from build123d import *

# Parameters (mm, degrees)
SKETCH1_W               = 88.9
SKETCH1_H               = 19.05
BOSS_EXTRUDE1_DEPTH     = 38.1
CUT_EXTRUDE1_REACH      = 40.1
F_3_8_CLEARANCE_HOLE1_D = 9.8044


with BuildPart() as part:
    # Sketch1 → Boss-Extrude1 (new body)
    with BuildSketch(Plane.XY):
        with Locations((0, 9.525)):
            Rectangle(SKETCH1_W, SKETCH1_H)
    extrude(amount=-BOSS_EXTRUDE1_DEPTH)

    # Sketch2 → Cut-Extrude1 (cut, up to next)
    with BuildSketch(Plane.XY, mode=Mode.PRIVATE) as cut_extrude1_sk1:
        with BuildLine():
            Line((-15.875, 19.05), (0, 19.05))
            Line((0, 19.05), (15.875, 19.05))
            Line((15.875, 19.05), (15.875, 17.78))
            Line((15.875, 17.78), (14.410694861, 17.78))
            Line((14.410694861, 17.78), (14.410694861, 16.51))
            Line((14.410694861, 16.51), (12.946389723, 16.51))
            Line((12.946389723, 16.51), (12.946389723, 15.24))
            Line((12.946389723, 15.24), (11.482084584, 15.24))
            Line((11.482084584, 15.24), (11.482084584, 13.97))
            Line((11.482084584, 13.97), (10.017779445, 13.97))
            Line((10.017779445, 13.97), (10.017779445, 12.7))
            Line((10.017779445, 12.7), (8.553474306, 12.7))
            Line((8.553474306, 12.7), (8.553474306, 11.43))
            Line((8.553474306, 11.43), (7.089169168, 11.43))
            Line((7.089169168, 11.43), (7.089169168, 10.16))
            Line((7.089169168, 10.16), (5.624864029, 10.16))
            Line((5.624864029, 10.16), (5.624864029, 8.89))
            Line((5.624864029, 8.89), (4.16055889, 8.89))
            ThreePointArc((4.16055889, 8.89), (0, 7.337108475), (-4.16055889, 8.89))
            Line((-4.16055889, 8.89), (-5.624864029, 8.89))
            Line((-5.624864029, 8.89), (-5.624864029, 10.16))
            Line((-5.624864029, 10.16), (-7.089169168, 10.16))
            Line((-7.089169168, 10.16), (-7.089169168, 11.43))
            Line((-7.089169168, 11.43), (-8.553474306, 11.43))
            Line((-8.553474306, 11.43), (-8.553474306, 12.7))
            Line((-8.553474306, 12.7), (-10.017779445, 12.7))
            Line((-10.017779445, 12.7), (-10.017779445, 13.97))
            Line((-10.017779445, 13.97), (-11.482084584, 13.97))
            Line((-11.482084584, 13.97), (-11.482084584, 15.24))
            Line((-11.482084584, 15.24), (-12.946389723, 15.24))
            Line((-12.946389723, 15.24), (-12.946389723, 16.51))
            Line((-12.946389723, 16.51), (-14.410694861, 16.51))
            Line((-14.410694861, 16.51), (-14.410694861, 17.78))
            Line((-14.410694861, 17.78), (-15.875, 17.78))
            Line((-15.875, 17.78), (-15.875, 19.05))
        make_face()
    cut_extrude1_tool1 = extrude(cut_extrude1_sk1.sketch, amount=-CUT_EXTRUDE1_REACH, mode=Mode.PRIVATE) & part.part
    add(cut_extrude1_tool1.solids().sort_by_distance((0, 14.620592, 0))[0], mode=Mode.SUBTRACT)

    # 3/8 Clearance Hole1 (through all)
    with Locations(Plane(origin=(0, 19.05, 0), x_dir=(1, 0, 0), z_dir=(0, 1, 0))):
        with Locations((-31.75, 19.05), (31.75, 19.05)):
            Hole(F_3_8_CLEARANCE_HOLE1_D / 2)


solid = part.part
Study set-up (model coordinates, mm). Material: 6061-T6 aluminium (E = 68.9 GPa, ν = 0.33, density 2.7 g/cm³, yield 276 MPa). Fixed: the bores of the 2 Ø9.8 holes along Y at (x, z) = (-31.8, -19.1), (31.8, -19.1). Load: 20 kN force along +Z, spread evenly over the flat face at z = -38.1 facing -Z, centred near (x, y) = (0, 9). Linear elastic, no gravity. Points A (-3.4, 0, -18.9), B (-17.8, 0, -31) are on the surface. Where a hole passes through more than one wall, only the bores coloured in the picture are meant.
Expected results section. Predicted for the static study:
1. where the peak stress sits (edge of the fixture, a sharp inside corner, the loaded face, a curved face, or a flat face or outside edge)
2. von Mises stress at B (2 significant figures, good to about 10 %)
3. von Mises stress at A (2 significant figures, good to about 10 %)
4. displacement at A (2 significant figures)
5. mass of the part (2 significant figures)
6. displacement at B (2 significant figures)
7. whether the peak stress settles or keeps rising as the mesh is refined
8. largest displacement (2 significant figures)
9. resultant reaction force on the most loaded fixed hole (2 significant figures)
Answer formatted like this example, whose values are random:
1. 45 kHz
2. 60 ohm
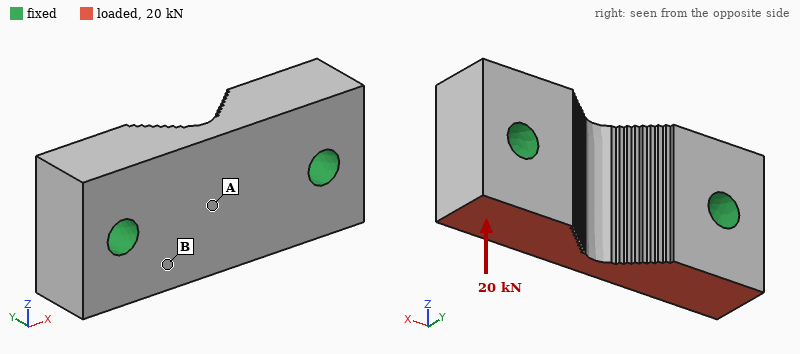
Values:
1. edge of the fixture
2. 18 MPa
3. 8.0 MPa
4. 12 µm
5. 140 g
6. 8.4 µm
7. keeps rising
8. 15 µm
9. 10 kN
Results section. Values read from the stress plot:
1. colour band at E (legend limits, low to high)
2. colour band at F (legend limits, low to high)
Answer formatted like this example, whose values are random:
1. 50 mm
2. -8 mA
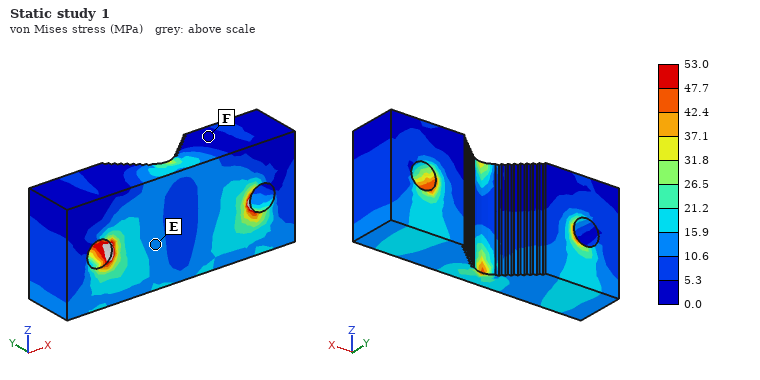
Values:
1. 10.6 to 15.9 MPa
2. 0.0 to 5.3 MPa
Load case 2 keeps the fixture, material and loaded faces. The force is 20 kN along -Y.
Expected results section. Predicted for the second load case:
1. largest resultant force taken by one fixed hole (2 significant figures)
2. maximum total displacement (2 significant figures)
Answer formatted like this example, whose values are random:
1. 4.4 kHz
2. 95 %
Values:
1. 10 kN
2. 58 µm
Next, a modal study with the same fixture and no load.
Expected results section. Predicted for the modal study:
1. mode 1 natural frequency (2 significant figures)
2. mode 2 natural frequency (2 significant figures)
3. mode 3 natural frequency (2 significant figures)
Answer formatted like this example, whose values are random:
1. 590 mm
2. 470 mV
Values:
1. 17 kHz
2. 18 kHz
3. 22 kHz
